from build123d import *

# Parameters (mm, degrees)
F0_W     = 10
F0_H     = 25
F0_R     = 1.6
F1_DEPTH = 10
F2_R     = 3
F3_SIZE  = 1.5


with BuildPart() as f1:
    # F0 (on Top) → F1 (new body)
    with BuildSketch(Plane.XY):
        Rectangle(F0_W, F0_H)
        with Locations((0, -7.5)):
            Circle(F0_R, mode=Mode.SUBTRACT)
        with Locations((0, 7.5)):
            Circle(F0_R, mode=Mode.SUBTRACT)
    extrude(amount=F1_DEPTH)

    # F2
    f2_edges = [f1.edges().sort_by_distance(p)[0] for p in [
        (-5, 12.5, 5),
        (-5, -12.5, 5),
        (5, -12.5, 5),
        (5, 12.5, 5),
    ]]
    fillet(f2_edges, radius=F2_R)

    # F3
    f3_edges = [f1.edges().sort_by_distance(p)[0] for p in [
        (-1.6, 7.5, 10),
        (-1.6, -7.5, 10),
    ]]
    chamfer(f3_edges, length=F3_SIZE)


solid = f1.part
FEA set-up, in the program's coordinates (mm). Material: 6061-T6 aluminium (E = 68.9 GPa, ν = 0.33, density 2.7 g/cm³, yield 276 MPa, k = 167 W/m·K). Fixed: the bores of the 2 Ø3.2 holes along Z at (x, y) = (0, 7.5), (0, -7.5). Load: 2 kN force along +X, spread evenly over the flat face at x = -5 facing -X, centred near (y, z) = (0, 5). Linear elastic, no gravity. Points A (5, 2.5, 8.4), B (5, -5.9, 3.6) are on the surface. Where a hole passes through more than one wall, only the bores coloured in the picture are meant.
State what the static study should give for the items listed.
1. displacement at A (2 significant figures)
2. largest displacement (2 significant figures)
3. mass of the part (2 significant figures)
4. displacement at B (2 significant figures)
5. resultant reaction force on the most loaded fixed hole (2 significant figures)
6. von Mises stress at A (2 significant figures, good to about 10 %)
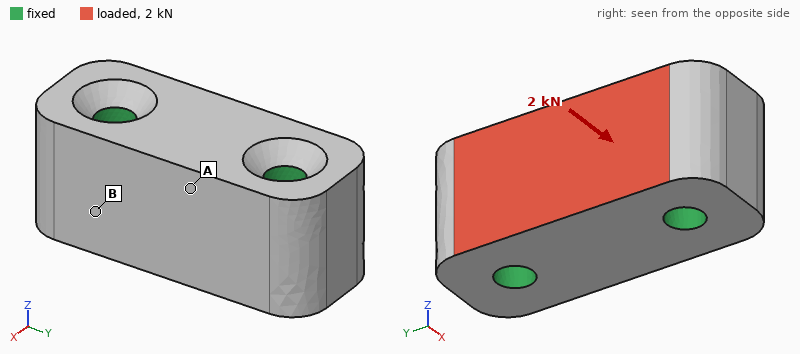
1.4 µm
2.5 µm
6.0 g
0.62 µm
1.0 kN
8.6 MPa
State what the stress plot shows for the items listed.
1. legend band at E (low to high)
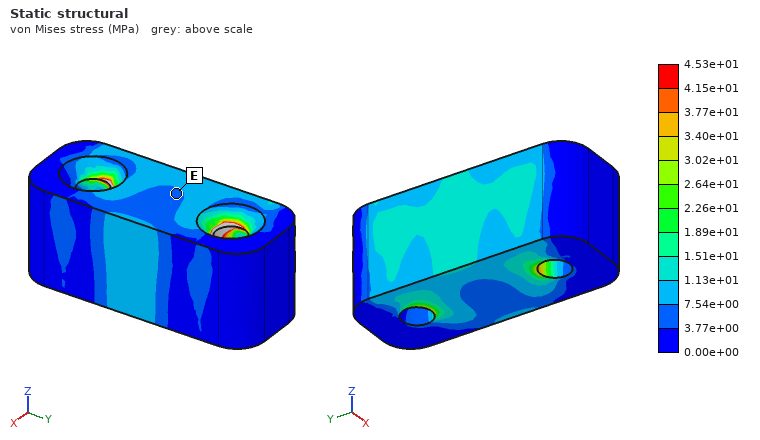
3.77e+00 to 7.54e+00 MPa
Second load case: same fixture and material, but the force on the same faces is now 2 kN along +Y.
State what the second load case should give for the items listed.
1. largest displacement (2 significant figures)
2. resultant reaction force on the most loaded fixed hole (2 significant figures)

2.2 µm
1.1 kN
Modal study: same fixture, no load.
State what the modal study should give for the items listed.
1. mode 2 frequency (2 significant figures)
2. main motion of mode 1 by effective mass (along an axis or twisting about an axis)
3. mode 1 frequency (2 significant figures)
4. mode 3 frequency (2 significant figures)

87 kHz
along X
80 kHz
88 kHz
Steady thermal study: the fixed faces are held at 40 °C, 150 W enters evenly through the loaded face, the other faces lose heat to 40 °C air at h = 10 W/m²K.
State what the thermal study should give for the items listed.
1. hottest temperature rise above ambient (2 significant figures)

31 K
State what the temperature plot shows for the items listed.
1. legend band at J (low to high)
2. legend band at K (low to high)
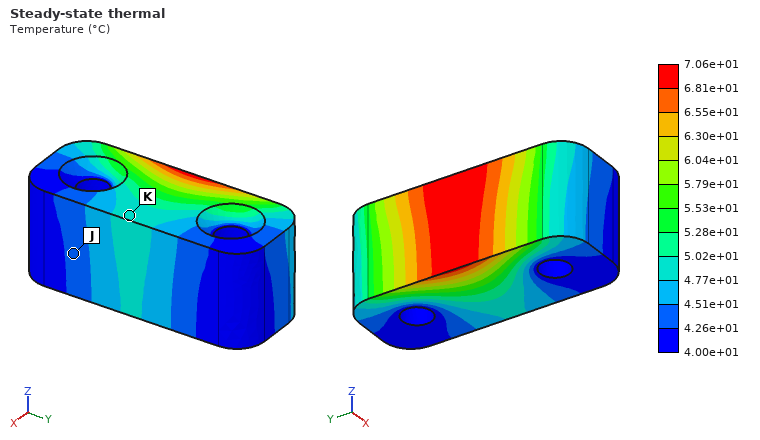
4.26e+01 to 4.51e+01 °C
4.77e+01 to 5.02e+01 °C
